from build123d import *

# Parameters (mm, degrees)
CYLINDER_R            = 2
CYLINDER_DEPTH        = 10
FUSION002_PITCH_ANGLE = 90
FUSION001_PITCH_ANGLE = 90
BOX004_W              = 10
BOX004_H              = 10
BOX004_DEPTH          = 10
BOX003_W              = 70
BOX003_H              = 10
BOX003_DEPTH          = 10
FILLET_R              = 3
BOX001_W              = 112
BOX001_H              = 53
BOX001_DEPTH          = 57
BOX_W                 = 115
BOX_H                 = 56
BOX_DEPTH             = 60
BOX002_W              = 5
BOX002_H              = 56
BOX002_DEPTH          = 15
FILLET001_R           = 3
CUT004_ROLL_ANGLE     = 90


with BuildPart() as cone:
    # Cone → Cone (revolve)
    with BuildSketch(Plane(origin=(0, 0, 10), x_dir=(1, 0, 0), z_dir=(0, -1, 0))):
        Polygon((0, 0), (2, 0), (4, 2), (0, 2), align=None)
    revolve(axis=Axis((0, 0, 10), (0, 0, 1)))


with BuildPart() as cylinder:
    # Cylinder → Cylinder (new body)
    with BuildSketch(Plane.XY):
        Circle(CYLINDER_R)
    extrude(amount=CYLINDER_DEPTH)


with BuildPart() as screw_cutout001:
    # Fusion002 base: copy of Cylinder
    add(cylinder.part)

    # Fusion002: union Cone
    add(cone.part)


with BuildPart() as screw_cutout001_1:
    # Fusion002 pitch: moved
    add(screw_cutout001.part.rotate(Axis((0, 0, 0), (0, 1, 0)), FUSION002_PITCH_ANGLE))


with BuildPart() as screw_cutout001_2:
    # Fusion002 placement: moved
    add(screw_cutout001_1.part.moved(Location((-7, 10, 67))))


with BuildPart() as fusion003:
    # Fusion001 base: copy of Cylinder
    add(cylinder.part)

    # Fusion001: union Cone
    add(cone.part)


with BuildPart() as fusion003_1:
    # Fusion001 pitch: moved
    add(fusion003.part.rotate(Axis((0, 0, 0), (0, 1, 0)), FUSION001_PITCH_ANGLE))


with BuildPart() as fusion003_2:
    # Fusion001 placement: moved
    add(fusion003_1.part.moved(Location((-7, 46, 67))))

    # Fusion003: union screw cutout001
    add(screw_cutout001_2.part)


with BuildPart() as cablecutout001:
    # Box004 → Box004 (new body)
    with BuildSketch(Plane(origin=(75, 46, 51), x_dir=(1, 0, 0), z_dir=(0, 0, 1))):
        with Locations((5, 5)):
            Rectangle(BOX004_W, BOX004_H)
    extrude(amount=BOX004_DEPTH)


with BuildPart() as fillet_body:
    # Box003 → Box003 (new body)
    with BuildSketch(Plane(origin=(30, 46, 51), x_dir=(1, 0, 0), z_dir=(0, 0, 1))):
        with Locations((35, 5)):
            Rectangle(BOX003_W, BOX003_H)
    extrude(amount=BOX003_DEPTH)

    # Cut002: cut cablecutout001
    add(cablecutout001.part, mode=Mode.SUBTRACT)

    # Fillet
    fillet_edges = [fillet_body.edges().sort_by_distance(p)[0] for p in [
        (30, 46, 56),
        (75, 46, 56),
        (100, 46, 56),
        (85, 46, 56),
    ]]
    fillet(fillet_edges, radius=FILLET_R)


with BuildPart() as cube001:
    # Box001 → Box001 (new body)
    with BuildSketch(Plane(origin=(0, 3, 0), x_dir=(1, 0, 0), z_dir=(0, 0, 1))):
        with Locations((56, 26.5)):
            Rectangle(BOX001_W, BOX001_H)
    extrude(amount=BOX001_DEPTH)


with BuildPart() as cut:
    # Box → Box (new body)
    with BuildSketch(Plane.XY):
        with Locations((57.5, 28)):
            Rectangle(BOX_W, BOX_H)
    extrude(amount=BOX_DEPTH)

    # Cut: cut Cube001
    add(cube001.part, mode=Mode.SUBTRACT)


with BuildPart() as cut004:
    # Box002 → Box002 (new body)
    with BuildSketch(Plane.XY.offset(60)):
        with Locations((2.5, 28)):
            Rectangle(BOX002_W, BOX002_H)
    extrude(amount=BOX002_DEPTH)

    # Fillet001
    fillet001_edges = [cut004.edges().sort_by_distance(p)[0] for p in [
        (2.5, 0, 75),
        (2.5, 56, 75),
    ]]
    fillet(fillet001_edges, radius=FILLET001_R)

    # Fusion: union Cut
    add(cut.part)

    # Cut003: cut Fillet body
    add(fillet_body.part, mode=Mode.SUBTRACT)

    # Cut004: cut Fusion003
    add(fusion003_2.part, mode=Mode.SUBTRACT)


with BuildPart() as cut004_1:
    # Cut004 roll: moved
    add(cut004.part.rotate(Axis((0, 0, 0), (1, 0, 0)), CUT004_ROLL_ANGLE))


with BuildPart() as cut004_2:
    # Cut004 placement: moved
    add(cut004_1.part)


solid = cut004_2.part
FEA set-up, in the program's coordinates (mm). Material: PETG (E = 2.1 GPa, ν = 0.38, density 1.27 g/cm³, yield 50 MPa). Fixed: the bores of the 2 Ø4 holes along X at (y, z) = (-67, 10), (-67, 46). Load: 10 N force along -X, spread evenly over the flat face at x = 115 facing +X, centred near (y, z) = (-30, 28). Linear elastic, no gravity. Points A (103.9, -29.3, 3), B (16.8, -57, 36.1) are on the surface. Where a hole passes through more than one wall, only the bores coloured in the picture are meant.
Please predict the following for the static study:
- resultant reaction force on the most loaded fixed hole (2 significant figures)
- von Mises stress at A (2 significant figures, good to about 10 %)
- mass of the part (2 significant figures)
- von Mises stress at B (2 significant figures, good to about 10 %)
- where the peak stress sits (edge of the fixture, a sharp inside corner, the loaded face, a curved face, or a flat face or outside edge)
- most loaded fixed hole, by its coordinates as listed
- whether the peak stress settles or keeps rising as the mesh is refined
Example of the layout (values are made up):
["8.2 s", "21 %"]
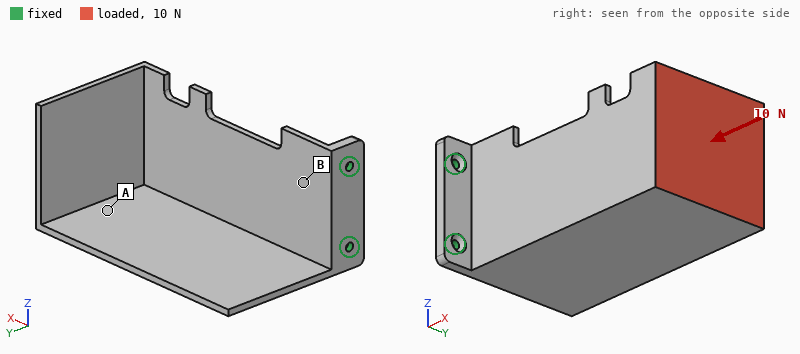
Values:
["5.5 N", "0.53 MPa", "64 g", "1.1 MPa", "edge of the fixture", "(-67, 10)", "keeps rising"]
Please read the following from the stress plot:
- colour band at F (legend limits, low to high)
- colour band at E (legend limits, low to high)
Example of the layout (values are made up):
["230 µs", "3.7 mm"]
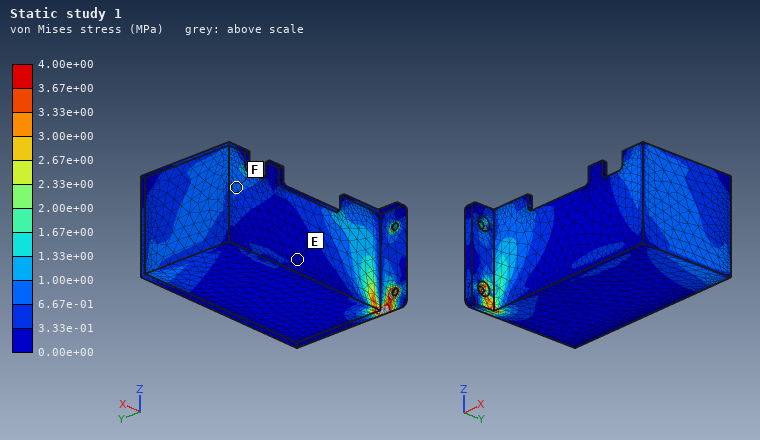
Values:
["6.67e-01 to 1.00e+00 MPa", "0.00e+00 to 3.33e-01 MPa"]
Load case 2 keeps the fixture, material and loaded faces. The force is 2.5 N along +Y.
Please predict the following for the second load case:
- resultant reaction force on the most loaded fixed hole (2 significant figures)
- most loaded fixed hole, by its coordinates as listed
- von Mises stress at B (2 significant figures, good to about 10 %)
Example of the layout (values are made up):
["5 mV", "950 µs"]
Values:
["2.2 N", "(-67, 46)", "1.0 MPa"]
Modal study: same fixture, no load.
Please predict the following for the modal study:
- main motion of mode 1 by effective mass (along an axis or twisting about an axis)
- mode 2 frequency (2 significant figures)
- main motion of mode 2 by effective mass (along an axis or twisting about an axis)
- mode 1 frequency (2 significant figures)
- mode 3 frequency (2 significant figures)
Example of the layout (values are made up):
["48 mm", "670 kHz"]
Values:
["along Y", "69 Hz", "along Z", "41 Hz", "210 Hz"]
